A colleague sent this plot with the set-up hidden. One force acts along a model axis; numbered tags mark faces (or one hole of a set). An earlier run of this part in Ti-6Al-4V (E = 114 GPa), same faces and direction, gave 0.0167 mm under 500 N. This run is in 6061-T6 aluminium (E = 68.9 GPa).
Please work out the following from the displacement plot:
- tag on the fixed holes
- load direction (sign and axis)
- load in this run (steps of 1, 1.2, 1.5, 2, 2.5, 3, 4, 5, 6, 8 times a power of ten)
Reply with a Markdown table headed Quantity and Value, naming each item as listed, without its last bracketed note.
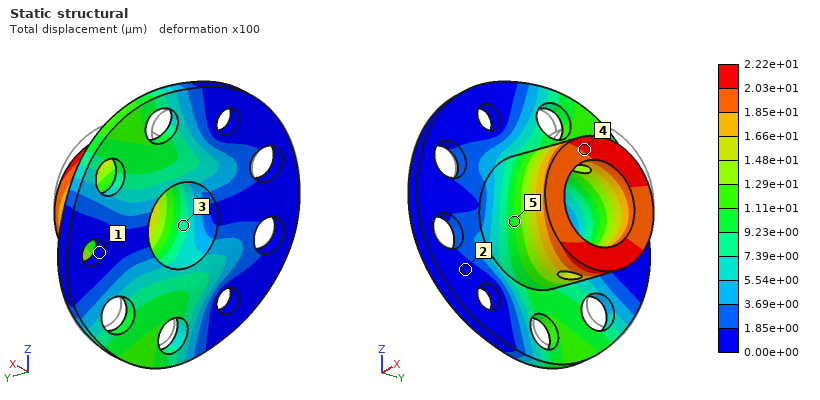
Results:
| Quantity | Value |
|---|---|
| tag on the fixed holes | 1 |
| load direction | -Z |
| load in this run | 400 N |
